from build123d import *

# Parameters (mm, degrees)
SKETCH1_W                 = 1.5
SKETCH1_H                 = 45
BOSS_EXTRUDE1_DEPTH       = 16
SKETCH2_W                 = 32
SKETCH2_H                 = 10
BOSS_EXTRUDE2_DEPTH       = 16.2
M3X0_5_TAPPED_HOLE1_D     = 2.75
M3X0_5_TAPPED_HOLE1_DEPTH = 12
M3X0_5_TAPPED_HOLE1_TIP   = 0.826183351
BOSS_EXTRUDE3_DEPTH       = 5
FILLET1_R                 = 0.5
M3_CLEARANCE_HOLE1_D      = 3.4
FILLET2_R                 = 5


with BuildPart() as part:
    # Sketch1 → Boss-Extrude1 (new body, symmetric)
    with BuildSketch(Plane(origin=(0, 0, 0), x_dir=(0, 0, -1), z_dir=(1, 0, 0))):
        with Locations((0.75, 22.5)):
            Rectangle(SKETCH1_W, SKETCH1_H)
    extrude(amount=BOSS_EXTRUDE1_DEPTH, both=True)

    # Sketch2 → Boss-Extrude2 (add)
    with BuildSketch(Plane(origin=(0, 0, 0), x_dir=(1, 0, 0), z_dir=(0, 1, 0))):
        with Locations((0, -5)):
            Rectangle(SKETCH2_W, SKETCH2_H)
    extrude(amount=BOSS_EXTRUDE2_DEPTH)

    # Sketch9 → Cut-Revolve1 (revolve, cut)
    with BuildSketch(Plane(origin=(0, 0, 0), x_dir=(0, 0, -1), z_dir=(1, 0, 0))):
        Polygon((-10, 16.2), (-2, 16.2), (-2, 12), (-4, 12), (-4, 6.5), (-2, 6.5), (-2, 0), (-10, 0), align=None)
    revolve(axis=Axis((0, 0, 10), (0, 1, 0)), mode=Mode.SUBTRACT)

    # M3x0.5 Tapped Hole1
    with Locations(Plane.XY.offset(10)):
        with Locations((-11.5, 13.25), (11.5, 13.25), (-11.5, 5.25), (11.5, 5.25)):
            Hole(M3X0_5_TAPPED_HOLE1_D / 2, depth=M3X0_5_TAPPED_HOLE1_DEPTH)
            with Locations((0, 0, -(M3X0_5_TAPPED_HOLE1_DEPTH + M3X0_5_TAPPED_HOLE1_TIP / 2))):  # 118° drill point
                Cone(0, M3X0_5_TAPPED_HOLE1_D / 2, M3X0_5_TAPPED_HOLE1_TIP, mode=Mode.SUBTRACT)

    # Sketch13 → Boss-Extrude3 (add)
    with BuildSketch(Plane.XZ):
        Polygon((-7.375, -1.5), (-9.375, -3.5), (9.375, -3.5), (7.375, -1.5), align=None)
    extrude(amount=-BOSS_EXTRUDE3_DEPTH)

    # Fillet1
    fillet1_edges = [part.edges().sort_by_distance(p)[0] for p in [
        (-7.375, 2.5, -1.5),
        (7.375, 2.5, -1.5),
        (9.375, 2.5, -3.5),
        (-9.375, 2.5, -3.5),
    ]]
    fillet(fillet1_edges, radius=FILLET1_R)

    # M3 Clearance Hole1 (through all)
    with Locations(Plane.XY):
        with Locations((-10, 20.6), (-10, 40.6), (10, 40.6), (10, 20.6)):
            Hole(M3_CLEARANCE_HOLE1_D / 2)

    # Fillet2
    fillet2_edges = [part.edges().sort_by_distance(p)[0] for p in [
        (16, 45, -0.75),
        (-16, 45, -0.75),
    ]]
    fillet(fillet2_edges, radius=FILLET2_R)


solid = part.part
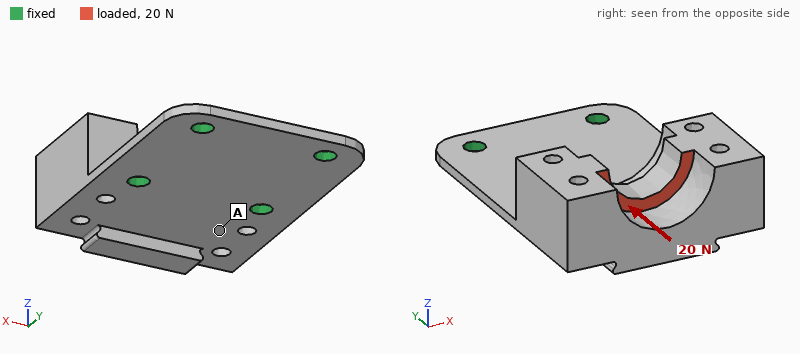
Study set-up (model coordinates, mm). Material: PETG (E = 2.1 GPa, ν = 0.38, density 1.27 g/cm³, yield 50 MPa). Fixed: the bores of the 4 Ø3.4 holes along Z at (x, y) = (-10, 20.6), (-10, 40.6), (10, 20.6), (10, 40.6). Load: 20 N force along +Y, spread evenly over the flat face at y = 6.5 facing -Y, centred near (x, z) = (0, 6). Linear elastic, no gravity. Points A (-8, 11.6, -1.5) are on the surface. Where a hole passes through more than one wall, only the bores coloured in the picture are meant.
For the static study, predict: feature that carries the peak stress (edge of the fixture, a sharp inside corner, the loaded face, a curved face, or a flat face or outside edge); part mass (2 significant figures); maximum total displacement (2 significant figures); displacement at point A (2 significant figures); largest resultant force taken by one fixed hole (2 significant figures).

a flat face or outside edge
7.3 g
0.58 mm
0.17 mm
8.6 N
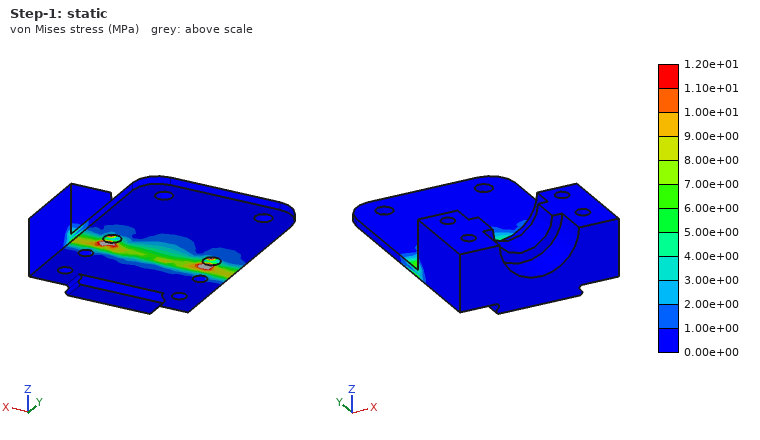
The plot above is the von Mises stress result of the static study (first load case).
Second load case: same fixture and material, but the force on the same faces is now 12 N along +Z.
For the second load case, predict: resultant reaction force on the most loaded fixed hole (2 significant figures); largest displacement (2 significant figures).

6.6 N
0.63 mm
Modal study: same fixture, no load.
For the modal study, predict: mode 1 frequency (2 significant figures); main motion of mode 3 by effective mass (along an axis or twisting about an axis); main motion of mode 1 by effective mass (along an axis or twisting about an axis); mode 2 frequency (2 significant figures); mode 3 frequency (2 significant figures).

370 Hz
along X
along Z
1700 Hz
3200 Hz
